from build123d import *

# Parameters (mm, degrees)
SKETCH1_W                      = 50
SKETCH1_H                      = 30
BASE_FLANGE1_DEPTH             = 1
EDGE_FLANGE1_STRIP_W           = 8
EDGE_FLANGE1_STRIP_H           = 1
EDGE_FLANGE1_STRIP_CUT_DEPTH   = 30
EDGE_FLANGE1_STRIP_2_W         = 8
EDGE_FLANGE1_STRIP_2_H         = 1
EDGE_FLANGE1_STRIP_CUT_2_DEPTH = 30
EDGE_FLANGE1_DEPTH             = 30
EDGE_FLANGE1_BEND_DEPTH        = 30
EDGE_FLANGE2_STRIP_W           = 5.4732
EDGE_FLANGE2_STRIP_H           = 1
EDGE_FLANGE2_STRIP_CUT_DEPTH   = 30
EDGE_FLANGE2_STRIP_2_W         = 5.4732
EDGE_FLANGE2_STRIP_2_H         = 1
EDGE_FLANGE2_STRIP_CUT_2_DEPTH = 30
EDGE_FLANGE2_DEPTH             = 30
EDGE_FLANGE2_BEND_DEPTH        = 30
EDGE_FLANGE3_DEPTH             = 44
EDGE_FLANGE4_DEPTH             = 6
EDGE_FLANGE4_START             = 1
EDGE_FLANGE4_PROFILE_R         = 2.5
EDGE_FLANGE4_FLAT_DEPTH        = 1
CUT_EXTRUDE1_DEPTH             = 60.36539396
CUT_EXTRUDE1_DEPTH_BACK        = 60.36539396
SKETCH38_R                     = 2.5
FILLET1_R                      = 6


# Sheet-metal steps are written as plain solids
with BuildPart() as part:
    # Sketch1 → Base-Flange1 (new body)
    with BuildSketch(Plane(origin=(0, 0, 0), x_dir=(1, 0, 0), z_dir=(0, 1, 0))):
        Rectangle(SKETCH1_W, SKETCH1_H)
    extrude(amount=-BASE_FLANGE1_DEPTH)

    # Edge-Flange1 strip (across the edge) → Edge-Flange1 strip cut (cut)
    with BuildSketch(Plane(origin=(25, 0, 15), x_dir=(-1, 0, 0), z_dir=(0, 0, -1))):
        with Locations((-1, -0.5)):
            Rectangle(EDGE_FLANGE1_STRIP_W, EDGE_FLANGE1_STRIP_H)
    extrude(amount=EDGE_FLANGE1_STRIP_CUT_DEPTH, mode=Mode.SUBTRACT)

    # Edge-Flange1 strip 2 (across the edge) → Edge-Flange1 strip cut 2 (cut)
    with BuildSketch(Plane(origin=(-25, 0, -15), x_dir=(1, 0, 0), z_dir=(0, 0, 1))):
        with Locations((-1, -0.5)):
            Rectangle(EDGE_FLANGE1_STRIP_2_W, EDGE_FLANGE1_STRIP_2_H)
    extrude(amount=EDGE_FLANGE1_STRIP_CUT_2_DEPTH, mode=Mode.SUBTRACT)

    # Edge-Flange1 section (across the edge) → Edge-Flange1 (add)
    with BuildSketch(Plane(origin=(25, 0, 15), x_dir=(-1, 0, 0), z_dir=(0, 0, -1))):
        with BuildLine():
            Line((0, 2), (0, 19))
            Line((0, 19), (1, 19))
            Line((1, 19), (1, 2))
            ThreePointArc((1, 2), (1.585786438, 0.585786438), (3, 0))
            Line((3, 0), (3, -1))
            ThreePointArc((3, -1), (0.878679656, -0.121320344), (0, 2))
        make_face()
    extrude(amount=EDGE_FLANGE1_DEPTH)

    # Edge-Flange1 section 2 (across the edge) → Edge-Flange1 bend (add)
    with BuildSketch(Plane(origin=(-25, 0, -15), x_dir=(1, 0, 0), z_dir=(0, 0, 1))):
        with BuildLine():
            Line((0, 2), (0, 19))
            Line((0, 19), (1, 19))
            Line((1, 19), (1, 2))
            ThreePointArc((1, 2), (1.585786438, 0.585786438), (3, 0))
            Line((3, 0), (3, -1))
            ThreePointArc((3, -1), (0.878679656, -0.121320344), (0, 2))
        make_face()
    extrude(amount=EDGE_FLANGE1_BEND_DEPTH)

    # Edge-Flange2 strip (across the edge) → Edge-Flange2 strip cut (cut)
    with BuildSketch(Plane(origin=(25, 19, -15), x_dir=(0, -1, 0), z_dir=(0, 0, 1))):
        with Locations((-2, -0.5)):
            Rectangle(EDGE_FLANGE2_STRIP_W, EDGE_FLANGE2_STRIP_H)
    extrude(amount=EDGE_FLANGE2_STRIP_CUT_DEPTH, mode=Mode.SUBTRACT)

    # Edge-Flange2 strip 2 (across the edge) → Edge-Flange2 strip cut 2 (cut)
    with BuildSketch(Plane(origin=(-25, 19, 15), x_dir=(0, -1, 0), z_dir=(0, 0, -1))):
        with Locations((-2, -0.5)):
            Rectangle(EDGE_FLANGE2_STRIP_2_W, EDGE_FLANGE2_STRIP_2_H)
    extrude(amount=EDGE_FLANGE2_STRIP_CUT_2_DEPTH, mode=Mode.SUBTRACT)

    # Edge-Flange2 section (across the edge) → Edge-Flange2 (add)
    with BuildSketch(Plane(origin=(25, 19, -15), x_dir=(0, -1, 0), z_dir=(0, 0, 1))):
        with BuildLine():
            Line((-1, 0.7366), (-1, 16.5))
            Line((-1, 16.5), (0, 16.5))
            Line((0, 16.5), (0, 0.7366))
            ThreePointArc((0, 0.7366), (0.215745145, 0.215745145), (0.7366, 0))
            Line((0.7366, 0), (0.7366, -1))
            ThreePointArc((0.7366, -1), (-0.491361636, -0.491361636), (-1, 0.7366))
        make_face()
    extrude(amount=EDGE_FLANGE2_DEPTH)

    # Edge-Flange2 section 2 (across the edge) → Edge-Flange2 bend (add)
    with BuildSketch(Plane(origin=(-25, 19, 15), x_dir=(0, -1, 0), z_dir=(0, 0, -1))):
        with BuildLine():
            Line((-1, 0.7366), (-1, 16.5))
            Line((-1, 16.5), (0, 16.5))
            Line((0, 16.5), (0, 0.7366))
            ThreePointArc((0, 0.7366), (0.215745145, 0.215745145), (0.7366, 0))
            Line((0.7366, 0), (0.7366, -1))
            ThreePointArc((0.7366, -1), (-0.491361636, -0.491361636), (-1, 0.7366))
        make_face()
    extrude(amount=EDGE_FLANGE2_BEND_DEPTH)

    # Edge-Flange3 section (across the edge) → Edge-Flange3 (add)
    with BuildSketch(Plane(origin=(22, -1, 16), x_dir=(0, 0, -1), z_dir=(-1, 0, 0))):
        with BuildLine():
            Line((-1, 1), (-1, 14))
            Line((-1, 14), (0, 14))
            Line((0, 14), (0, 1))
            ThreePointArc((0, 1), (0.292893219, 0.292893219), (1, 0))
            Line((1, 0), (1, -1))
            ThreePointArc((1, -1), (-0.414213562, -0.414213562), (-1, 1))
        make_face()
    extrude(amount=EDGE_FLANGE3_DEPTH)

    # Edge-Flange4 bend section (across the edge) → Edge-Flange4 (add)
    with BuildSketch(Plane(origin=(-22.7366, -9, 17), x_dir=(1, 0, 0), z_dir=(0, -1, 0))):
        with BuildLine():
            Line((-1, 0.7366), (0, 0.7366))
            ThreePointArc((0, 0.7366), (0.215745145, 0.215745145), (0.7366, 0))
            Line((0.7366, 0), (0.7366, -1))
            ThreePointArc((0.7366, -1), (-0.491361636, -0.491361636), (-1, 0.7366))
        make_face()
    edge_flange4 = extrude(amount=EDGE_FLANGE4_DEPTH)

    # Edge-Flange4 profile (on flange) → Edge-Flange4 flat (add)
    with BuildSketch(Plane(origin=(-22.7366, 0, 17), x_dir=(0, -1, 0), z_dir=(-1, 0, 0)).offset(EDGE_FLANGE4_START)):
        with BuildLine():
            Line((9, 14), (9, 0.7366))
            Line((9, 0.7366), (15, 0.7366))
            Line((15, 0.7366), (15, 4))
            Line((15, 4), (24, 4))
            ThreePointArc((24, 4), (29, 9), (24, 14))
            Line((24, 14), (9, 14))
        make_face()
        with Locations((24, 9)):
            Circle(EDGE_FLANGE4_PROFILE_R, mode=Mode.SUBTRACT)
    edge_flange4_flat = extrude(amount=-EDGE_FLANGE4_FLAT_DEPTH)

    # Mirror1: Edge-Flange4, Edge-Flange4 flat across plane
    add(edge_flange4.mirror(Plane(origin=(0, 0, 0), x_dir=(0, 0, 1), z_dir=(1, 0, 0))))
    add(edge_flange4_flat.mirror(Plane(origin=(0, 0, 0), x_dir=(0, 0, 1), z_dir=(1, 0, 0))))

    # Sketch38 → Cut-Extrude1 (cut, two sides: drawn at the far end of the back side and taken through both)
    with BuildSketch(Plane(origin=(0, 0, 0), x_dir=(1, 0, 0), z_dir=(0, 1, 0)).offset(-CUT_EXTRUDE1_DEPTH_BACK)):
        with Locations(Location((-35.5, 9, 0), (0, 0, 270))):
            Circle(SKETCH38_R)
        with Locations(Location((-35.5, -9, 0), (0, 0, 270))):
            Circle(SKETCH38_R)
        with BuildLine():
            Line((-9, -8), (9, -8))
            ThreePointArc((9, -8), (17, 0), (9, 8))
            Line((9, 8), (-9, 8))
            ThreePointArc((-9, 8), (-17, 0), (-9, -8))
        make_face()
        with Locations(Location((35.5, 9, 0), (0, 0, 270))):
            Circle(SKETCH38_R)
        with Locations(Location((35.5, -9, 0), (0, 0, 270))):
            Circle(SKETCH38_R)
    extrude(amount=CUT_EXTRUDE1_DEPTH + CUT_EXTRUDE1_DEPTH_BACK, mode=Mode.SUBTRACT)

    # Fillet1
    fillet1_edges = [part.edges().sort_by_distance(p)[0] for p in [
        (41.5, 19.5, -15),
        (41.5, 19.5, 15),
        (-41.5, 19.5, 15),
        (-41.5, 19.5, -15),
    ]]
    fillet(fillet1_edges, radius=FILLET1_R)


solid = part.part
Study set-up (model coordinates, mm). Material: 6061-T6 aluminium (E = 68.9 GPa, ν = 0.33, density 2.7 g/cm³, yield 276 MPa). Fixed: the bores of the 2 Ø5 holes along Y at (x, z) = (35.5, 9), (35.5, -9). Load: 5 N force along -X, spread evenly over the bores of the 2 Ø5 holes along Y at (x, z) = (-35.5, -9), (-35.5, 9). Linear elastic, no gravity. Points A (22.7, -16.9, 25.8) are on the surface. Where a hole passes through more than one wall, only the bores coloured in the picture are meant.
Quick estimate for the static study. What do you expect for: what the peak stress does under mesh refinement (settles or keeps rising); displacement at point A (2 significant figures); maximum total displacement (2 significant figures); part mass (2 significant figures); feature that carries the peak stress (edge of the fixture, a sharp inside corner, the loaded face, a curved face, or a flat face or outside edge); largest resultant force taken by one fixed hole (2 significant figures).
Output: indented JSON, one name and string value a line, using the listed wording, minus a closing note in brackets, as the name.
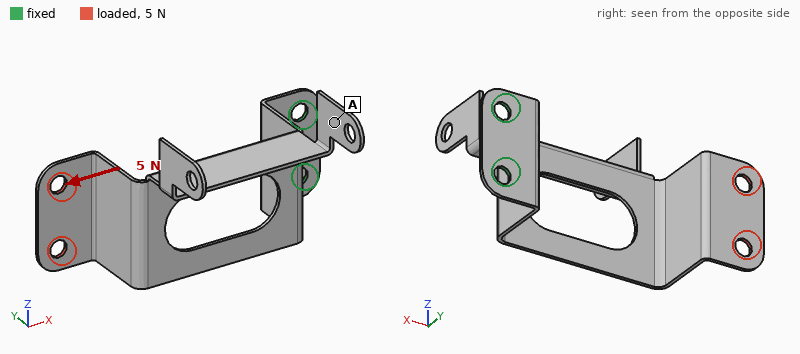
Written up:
{
  "what the peak stress does under mesh refinement": "keeps rising",
  "displacement at point A": "0.29 mm",
  "maximum total displacement": "1.3 mm",
  "part mass": "11 g",
  "feature that carries the peak stress": "a sharp inside corner",
  "largest resultant force taken by one fixed hole": "2.5 N"
}
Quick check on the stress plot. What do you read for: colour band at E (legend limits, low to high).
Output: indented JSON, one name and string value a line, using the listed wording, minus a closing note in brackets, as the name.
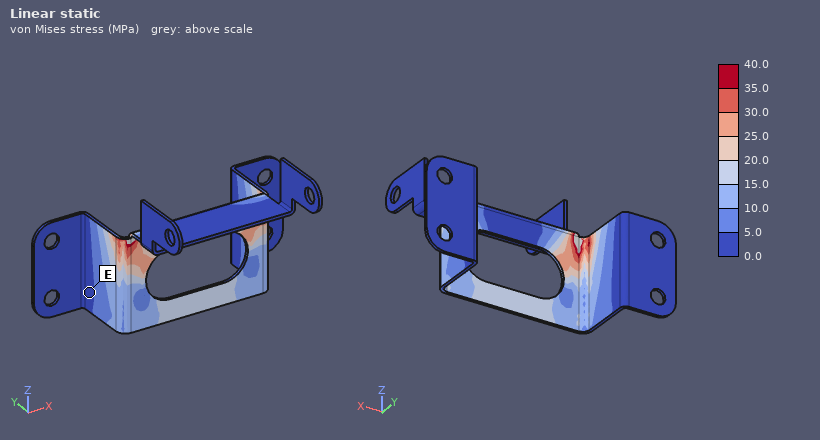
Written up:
{
  "colour band at E": "0.0 to 5.0 MPa"
}
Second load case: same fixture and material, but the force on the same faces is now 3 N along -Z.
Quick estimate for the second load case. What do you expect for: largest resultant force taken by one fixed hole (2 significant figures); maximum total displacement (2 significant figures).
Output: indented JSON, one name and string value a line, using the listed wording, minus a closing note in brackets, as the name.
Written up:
{
  "largest resultant force taken by one fixed hole": "10 N",
  "maximum total displacement": "1.00 mm"
}
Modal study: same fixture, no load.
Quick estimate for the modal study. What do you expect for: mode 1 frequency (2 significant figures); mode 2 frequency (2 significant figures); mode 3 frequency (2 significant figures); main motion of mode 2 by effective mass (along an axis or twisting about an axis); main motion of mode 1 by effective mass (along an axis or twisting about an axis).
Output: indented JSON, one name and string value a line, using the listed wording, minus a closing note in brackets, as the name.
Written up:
{
  "mode 1 frequency": "88 Hz",
  "mode 2 frequency": "180 Hz",
  "mode 3 frequency": "350 Hz",
  "main motion of mode 2 by effective mass": "along Z",
  "main motion of mode 1 by effective mass": "along Y"
}
